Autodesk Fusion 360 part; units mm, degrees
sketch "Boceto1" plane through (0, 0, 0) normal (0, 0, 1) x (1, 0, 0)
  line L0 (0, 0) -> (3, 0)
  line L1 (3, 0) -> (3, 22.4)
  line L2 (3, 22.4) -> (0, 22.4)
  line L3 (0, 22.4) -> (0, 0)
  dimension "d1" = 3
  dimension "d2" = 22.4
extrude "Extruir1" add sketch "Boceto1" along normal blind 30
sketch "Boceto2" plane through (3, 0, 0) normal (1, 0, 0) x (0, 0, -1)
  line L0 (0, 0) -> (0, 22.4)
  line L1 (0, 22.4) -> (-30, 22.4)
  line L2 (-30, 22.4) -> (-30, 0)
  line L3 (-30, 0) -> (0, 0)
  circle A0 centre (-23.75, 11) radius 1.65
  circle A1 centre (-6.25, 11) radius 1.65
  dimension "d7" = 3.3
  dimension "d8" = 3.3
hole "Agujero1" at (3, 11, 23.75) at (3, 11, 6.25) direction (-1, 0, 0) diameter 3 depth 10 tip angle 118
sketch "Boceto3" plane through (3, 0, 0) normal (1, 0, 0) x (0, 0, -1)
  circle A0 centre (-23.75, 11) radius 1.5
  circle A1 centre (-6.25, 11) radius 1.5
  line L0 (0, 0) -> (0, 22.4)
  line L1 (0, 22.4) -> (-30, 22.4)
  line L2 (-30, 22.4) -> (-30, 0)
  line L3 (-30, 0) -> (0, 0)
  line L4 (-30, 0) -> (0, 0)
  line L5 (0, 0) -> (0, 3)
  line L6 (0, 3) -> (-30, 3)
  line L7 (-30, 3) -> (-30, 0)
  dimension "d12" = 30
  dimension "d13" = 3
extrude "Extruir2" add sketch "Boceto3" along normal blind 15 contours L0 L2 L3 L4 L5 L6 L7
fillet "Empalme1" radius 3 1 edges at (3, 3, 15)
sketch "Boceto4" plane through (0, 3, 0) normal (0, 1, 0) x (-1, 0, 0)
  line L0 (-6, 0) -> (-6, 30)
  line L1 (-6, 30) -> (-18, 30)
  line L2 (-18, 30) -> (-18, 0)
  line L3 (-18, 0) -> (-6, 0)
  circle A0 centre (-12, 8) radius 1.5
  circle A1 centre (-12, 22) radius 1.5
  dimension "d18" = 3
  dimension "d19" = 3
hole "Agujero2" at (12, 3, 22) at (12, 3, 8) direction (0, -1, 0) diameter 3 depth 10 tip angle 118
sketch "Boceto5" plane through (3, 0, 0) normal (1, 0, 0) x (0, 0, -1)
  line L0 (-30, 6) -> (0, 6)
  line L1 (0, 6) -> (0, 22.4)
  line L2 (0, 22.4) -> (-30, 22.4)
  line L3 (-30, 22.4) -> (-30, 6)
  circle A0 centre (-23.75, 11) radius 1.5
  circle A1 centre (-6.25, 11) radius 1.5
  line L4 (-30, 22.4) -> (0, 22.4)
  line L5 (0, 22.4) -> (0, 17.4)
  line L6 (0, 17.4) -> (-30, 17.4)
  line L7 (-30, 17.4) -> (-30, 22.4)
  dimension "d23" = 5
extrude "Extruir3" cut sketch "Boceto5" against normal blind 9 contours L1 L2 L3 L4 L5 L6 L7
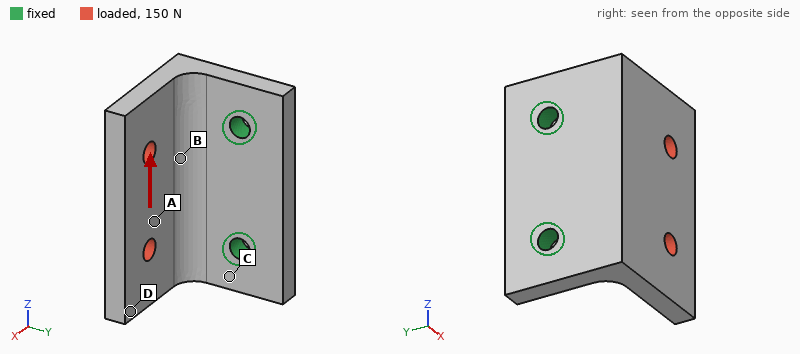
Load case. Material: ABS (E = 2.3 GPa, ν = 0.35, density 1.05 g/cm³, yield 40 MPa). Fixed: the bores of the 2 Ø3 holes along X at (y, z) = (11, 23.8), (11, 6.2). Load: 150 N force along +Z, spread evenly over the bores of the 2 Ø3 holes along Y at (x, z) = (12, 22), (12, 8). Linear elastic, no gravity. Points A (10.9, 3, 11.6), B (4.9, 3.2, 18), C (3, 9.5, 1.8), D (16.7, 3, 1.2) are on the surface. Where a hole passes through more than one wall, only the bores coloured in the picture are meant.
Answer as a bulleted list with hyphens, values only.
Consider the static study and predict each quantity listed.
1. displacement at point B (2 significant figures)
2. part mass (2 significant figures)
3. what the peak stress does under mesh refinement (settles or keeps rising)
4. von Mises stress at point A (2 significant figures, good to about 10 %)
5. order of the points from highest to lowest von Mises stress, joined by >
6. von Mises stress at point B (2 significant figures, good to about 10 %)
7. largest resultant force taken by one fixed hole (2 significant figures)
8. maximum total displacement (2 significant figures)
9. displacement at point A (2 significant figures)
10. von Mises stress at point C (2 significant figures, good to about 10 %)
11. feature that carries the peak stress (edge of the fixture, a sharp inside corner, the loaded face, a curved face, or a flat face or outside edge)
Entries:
- 0.079 mm
- 3.0 g
- keeps rising
- 6.5 MPa
- B > C > A > D
- 14 MPa
- 130 N
- 0.40 mm
- 0.19 mm
- 9.9 MPa
- edge of the fixture
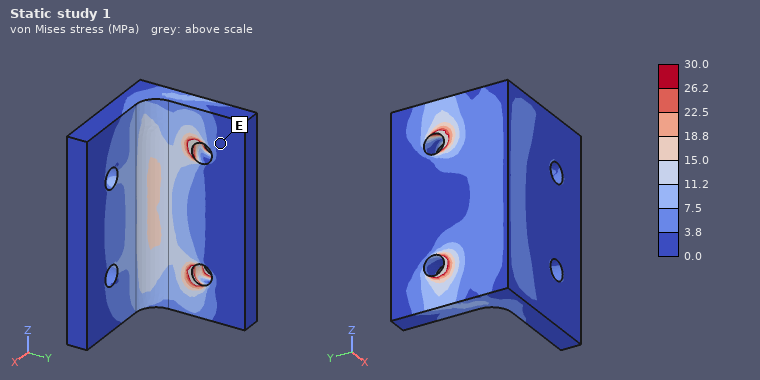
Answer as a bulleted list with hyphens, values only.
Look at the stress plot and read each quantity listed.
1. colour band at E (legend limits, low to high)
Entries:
- 0.0 to 3.8 MPa
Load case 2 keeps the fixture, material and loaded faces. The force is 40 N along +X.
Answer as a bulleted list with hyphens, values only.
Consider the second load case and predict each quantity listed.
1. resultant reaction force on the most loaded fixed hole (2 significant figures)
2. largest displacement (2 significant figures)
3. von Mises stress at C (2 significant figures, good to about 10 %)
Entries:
- 20 N
- 0.21 mm
- 4.2 MPa
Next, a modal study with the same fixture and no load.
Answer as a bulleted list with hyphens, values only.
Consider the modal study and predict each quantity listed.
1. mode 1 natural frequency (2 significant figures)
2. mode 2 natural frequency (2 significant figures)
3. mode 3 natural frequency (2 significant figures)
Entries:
- 1500 Hz
- 2700 Hz
- 4500 Hz
